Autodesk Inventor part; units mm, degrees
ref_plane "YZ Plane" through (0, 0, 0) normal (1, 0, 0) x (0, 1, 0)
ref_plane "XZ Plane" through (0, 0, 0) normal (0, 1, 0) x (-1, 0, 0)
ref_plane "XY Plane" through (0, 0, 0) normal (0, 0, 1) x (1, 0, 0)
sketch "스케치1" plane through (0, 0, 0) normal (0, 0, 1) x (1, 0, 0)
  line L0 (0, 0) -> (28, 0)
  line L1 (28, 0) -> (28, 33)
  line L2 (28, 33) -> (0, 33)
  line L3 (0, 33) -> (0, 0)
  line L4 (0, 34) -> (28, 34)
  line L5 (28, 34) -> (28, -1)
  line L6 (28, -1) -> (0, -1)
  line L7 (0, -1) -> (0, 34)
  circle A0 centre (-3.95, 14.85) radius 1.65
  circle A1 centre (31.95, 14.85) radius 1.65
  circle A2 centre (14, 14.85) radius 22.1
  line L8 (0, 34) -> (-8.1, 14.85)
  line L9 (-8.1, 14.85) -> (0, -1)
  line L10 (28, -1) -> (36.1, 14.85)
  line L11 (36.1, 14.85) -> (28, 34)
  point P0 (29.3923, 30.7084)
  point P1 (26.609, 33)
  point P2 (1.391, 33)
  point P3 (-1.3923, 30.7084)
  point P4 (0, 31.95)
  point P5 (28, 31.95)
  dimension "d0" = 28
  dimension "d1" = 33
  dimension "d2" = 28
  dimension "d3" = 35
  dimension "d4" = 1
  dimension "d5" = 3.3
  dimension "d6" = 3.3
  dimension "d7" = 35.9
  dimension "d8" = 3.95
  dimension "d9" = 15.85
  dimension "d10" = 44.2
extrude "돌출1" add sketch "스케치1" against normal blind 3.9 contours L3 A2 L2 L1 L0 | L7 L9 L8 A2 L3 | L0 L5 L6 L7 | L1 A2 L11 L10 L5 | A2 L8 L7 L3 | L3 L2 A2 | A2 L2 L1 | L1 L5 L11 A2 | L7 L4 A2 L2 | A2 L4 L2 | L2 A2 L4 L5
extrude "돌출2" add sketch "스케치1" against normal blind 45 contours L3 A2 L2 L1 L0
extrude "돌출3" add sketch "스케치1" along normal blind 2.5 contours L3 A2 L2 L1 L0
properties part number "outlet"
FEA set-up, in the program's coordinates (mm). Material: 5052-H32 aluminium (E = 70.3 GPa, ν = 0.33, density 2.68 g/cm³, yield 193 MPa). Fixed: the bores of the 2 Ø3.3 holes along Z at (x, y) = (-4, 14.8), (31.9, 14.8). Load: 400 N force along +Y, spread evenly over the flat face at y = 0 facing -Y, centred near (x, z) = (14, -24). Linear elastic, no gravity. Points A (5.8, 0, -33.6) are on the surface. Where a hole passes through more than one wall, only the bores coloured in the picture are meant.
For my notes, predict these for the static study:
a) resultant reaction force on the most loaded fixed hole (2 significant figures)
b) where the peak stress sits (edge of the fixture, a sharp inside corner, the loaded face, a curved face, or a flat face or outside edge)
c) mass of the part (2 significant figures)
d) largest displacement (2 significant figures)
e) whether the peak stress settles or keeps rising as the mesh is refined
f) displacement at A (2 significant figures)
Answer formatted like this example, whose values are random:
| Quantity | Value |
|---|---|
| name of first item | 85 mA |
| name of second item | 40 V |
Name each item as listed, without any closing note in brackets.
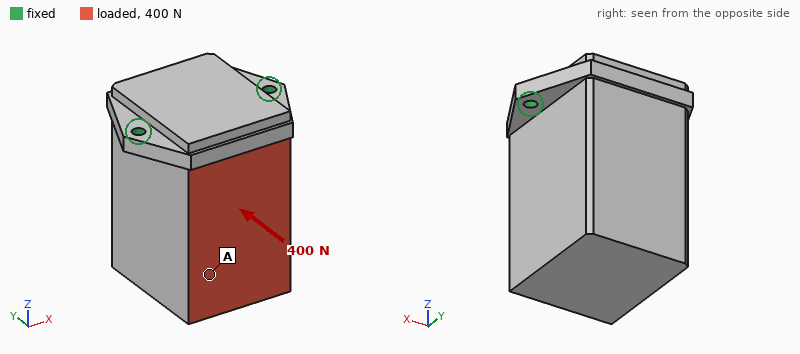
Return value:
| Quantity | Value |
|---|---|
| resultant reaction force on the most loaded fixed hole | 200 N |
| where the peak stress sits | edge of the fixture |
| mass of the part | 120 g |
| largest displacement | 0.11 mm |
| whether the peak stress settles or keeps rising as the mesh is refined | keeps rising |
| displacement at A | 0.085 mm |
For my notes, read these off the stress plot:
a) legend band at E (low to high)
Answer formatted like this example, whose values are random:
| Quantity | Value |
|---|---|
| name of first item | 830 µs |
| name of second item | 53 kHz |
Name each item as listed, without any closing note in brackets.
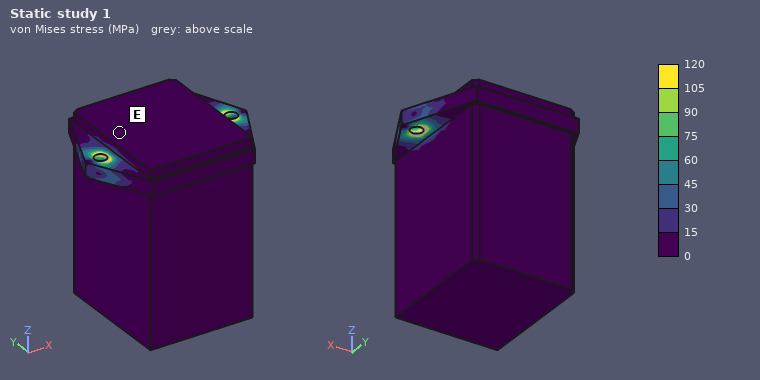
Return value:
| Quantity | Value |
|---|---|
| legend band at E | 0 to 15 MPa |
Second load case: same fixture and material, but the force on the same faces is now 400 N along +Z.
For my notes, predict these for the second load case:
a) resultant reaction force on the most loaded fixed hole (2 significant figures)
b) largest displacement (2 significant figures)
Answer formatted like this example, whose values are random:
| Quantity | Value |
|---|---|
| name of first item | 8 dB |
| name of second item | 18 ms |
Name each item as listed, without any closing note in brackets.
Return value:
| Quantity | Value |
|---|---|
| resultant reaction force on the most loaded fixed hole | 200 N |
| largest displacement | 73 µm |
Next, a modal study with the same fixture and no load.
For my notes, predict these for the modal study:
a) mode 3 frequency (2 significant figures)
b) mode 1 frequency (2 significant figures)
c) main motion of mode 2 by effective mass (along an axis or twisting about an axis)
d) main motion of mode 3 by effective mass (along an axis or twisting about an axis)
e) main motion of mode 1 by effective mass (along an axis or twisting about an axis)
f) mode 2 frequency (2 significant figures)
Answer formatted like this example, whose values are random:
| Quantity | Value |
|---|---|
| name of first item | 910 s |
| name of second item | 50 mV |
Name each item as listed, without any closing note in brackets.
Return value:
| Quantity | Value |
|---|---|
| mode 3 frequency | 7300 Hz |
| mode 1 frequency | 1100 Hz |
| main motion of mode 2 by effective mass | along X |
| main motion of mode 3 by effective mass | along Z |
| main motion of mode 1 by effective mass | along Y |
| mode 2 frequency | 4400 Hz |
